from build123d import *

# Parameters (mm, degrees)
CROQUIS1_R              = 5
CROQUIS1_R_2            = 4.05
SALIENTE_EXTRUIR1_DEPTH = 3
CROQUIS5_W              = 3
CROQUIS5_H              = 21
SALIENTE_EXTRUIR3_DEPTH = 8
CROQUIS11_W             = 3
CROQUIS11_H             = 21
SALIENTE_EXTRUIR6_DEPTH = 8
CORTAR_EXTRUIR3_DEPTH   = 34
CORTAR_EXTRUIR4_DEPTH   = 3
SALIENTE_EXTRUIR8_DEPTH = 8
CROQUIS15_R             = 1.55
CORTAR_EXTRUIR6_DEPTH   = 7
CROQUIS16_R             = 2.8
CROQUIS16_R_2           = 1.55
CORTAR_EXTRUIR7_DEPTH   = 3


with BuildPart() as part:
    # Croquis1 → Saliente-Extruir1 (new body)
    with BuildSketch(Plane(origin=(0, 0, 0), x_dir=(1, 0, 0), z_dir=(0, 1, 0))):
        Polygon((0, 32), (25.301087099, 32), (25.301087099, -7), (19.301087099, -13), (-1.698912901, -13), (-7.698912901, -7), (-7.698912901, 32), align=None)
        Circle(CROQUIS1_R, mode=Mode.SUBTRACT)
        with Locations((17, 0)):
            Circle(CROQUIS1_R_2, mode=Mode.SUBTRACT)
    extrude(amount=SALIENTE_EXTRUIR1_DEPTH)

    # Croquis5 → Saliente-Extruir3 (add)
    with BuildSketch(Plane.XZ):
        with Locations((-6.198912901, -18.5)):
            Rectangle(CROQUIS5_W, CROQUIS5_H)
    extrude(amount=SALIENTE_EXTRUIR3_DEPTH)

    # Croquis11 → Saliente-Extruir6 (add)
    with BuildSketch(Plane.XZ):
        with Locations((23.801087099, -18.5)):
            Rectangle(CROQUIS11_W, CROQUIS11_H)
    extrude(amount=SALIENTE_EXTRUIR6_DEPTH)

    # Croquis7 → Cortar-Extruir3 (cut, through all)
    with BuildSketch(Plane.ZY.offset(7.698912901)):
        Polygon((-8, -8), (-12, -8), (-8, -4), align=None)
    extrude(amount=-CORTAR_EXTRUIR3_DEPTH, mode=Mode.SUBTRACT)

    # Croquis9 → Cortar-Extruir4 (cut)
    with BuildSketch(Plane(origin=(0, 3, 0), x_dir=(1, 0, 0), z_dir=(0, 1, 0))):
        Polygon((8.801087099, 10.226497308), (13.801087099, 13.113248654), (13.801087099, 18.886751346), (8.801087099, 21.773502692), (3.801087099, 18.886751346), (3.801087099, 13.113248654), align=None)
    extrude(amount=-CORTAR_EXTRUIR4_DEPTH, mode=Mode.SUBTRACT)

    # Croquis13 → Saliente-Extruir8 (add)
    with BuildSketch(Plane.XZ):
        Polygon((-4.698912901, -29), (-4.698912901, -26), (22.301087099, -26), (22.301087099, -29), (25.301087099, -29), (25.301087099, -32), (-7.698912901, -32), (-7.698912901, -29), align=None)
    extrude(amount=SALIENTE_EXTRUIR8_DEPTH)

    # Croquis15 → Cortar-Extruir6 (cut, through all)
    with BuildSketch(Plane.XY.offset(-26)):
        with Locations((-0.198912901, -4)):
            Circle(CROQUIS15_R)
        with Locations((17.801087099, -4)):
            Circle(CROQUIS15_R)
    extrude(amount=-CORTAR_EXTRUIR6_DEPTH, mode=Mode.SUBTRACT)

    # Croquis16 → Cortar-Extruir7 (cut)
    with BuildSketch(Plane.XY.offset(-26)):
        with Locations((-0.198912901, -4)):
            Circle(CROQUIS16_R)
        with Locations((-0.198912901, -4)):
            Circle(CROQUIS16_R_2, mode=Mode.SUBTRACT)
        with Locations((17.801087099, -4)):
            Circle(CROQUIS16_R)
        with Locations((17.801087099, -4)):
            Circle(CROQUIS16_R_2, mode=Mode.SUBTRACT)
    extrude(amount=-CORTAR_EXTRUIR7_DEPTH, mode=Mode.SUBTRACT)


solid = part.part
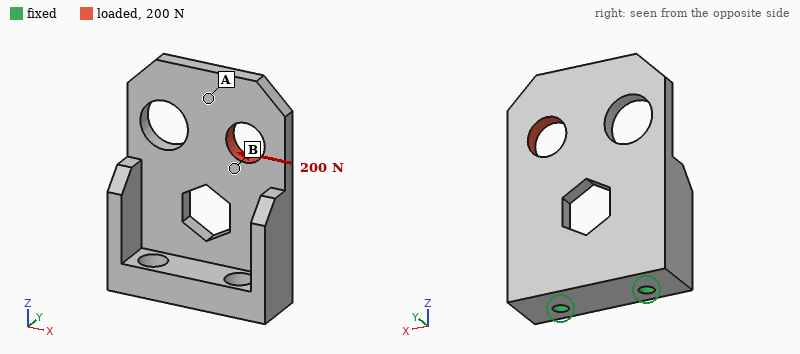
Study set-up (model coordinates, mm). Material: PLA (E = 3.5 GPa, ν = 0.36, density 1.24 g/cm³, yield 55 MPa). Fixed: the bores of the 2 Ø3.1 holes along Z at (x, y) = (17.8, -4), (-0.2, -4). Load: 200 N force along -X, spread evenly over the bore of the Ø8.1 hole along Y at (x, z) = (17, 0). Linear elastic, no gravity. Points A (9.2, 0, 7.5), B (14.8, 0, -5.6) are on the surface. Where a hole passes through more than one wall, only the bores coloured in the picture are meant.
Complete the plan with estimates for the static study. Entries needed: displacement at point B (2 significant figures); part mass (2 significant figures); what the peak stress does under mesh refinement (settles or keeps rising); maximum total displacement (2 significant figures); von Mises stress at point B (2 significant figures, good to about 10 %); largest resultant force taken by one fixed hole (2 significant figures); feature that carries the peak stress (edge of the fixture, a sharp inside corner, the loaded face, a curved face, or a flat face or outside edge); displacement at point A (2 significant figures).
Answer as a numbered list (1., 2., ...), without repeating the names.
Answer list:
1. 0.31 mm
2. 7.3 g
3. keeps rising
4. 0.56 mm
5. 13 MPa
6. 320 N
7. edge of the fixture
8. 0.43 mm
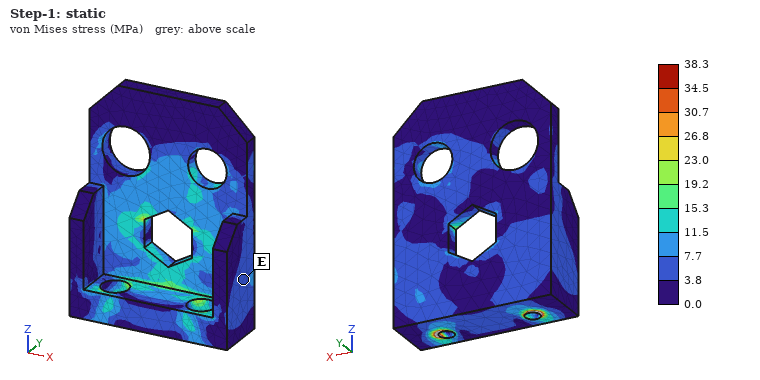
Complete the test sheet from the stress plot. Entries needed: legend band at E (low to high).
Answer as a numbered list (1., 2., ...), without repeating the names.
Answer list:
1. 3.8 to 7.7 MPa
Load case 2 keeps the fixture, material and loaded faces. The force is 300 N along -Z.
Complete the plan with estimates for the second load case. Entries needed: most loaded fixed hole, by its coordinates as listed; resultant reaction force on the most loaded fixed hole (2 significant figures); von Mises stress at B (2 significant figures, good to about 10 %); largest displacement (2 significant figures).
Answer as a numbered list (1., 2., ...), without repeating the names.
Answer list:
1. (17.8, -4)
2. 270 N
3. 8.5 MPa
4. 0.65 mm
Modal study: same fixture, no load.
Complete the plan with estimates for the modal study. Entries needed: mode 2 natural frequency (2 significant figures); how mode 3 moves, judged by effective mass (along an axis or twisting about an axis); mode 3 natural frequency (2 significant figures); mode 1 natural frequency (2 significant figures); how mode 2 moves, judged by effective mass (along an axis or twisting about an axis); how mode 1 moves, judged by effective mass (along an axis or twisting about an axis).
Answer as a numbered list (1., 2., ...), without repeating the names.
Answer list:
1. 1600 Hz
2. along Y
3. 2500 Hz
4. 760 Hz
5. along X
6. along Y
